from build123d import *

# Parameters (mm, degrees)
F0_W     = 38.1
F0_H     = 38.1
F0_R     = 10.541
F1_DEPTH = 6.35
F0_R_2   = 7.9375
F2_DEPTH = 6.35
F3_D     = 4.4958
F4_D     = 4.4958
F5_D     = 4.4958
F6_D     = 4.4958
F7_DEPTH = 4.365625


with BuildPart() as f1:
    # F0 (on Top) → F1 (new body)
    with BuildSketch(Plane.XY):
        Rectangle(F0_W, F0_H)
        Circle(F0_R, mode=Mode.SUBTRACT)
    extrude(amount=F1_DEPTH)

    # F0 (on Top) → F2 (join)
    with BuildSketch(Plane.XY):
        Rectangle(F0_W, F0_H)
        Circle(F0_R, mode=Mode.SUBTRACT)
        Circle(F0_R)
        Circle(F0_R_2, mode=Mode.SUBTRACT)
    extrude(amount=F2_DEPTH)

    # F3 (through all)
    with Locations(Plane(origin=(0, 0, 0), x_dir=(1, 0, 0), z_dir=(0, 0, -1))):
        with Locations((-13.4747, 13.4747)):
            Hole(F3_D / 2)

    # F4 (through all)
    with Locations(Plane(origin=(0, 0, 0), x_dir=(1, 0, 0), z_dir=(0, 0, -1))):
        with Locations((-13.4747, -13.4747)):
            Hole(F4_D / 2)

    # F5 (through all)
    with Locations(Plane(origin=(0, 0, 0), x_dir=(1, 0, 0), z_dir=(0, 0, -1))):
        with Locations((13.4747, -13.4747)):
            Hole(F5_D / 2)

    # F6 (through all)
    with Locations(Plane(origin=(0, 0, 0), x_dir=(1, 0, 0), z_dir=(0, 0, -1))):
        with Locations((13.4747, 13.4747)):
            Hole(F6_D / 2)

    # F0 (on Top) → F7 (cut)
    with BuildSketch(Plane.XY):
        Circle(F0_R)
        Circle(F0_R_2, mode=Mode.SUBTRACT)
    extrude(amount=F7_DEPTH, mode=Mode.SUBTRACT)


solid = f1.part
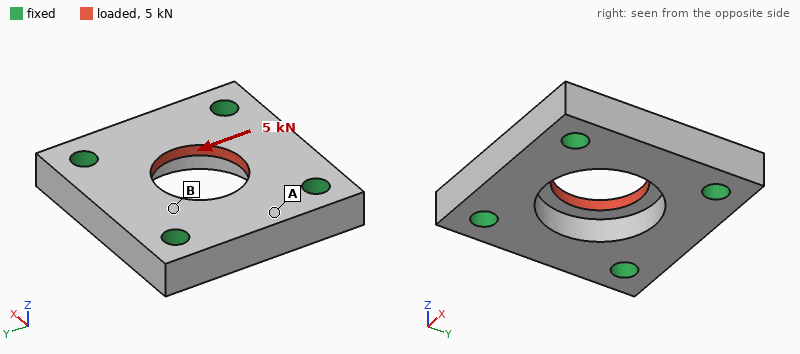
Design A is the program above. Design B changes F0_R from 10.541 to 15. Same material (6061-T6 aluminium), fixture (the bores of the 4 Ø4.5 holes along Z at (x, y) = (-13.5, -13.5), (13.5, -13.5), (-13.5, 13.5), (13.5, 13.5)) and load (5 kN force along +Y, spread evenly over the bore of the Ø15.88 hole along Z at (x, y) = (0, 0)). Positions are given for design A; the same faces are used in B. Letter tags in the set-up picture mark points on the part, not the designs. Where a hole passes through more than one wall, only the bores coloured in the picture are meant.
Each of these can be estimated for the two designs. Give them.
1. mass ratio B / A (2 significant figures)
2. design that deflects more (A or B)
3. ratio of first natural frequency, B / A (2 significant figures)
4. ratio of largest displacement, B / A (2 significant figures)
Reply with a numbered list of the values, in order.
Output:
1. 0.77
2. B
3. 0.71
4. 1.2
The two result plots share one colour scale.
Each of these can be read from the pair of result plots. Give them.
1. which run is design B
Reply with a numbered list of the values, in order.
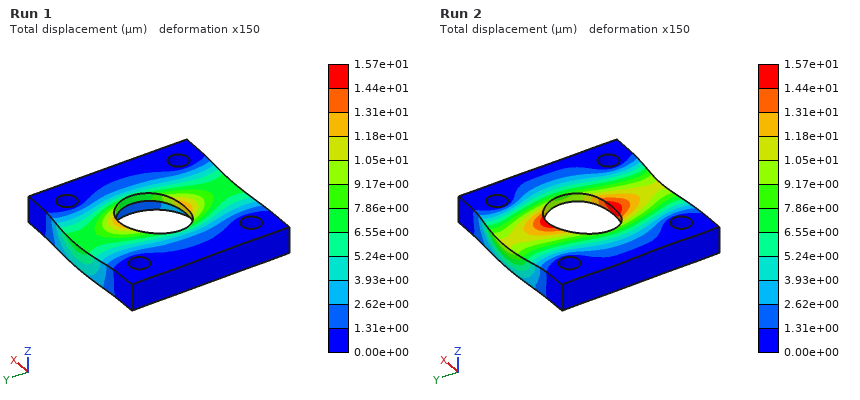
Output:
1. Run 2
